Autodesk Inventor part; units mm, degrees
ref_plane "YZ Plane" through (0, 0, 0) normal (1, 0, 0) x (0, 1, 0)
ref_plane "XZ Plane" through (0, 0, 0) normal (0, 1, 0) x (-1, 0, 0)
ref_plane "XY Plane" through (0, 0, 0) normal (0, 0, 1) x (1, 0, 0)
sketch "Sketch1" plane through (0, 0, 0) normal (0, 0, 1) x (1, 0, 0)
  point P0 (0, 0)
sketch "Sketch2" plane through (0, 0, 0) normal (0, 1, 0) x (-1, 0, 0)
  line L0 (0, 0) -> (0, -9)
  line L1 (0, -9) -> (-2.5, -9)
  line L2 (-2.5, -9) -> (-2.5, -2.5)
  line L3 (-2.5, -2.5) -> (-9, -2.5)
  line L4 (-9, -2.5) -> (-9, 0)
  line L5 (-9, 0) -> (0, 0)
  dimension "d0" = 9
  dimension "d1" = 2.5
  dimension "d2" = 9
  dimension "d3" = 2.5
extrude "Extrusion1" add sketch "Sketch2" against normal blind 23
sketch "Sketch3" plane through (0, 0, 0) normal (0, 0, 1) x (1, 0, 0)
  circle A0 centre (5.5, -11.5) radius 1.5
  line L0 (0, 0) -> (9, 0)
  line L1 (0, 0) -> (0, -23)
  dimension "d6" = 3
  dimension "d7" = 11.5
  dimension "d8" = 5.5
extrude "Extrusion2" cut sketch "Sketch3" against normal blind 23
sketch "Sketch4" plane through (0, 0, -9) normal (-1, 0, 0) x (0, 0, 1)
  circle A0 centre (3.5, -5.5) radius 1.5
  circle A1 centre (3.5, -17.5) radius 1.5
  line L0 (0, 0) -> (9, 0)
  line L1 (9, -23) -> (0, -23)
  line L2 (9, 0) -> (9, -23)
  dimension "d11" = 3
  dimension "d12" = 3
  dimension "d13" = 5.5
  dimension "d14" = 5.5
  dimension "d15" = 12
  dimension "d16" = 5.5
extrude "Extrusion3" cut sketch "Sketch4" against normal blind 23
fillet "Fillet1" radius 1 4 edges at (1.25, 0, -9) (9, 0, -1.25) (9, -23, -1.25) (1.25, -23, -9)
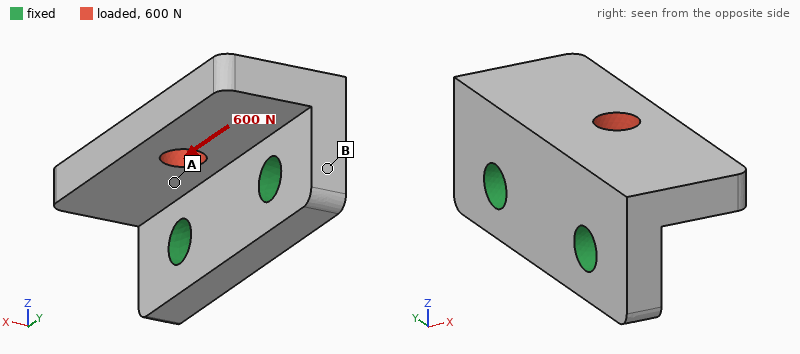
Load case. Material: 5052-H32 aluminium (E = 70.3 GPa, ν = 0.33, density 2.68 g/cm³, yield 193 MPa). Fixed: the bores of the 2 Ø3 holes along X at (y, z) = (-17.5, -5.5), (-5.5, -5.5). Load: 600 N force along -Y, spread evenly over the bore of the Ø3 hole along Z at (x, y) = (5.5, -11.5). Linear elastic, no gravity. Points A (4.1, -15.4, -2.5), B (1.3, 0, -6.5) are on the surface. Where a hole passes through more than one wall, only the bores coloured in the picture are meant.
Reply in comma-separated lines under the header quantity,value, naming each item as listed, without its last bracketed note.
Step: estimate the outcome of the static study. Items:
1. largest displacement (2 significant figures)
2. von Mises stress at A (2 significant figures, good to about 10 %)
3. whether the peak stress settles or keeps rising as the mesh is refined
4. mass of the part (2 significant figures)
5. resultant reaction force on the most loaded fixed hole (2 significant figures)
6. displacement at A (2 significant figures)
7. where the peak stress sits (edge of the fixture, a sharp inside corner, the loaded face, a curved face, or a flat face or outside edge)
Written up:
quantity,value
largest displacement,12 µm
von Mises stress at A,36 MPa
whether the peak stress settles or keeps rising as the mesh is refined,keeps rising
mass of the part,2.2 g
resultant reaction force on the most loaded fixed hole,380 N
displacement at A,4.6 µm
where the peak stress sits,edge of the fixture
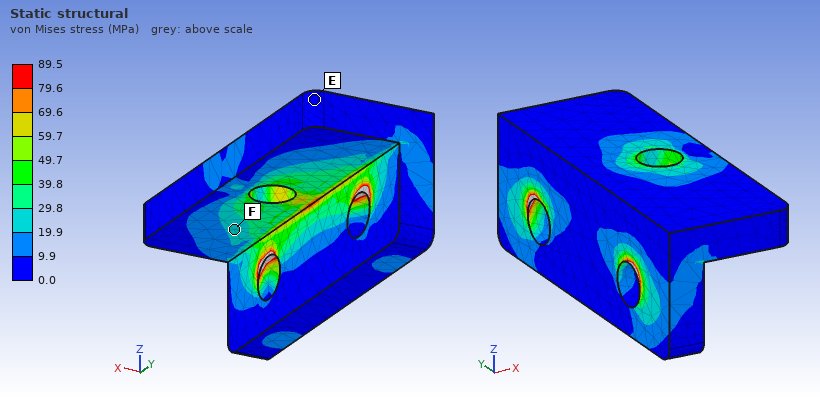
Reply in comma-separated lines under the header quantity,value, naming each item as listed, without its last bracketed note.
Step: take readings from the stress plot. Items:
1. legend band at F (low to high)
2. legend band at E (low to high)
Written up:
quantity,value
legend band at F,19.9 to 29.8 MPa
legend band at E,0.0 to 9.9 MPa
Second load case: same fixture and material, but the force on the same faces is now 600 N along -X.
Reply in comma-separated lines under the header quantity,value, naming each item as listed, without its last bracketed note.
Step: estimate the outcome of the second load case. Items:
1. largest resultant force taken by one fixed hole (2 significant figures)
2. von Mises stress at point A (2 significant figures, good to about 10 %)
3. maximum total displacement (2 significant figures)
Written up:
quantity,value
largest resultant force taken by one fixed hole,310 N
von Mises stress at point A,26 MPa
maximum total displacement,24 µm
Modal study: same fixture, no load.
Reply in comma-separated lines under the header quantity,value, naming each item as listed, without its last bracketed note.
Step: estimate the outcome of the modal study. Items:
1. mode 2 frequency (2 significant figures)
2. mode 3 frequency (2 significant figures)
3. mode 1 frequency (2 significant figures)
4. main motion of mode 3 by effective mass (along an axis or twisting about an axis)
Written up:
quantity,value
mode 2 frequency,26 kHz
mode 3 frequency,43 kHz
mode 1 frequency,20 kHz
main motion of mode 3 by effective mass,along Y
